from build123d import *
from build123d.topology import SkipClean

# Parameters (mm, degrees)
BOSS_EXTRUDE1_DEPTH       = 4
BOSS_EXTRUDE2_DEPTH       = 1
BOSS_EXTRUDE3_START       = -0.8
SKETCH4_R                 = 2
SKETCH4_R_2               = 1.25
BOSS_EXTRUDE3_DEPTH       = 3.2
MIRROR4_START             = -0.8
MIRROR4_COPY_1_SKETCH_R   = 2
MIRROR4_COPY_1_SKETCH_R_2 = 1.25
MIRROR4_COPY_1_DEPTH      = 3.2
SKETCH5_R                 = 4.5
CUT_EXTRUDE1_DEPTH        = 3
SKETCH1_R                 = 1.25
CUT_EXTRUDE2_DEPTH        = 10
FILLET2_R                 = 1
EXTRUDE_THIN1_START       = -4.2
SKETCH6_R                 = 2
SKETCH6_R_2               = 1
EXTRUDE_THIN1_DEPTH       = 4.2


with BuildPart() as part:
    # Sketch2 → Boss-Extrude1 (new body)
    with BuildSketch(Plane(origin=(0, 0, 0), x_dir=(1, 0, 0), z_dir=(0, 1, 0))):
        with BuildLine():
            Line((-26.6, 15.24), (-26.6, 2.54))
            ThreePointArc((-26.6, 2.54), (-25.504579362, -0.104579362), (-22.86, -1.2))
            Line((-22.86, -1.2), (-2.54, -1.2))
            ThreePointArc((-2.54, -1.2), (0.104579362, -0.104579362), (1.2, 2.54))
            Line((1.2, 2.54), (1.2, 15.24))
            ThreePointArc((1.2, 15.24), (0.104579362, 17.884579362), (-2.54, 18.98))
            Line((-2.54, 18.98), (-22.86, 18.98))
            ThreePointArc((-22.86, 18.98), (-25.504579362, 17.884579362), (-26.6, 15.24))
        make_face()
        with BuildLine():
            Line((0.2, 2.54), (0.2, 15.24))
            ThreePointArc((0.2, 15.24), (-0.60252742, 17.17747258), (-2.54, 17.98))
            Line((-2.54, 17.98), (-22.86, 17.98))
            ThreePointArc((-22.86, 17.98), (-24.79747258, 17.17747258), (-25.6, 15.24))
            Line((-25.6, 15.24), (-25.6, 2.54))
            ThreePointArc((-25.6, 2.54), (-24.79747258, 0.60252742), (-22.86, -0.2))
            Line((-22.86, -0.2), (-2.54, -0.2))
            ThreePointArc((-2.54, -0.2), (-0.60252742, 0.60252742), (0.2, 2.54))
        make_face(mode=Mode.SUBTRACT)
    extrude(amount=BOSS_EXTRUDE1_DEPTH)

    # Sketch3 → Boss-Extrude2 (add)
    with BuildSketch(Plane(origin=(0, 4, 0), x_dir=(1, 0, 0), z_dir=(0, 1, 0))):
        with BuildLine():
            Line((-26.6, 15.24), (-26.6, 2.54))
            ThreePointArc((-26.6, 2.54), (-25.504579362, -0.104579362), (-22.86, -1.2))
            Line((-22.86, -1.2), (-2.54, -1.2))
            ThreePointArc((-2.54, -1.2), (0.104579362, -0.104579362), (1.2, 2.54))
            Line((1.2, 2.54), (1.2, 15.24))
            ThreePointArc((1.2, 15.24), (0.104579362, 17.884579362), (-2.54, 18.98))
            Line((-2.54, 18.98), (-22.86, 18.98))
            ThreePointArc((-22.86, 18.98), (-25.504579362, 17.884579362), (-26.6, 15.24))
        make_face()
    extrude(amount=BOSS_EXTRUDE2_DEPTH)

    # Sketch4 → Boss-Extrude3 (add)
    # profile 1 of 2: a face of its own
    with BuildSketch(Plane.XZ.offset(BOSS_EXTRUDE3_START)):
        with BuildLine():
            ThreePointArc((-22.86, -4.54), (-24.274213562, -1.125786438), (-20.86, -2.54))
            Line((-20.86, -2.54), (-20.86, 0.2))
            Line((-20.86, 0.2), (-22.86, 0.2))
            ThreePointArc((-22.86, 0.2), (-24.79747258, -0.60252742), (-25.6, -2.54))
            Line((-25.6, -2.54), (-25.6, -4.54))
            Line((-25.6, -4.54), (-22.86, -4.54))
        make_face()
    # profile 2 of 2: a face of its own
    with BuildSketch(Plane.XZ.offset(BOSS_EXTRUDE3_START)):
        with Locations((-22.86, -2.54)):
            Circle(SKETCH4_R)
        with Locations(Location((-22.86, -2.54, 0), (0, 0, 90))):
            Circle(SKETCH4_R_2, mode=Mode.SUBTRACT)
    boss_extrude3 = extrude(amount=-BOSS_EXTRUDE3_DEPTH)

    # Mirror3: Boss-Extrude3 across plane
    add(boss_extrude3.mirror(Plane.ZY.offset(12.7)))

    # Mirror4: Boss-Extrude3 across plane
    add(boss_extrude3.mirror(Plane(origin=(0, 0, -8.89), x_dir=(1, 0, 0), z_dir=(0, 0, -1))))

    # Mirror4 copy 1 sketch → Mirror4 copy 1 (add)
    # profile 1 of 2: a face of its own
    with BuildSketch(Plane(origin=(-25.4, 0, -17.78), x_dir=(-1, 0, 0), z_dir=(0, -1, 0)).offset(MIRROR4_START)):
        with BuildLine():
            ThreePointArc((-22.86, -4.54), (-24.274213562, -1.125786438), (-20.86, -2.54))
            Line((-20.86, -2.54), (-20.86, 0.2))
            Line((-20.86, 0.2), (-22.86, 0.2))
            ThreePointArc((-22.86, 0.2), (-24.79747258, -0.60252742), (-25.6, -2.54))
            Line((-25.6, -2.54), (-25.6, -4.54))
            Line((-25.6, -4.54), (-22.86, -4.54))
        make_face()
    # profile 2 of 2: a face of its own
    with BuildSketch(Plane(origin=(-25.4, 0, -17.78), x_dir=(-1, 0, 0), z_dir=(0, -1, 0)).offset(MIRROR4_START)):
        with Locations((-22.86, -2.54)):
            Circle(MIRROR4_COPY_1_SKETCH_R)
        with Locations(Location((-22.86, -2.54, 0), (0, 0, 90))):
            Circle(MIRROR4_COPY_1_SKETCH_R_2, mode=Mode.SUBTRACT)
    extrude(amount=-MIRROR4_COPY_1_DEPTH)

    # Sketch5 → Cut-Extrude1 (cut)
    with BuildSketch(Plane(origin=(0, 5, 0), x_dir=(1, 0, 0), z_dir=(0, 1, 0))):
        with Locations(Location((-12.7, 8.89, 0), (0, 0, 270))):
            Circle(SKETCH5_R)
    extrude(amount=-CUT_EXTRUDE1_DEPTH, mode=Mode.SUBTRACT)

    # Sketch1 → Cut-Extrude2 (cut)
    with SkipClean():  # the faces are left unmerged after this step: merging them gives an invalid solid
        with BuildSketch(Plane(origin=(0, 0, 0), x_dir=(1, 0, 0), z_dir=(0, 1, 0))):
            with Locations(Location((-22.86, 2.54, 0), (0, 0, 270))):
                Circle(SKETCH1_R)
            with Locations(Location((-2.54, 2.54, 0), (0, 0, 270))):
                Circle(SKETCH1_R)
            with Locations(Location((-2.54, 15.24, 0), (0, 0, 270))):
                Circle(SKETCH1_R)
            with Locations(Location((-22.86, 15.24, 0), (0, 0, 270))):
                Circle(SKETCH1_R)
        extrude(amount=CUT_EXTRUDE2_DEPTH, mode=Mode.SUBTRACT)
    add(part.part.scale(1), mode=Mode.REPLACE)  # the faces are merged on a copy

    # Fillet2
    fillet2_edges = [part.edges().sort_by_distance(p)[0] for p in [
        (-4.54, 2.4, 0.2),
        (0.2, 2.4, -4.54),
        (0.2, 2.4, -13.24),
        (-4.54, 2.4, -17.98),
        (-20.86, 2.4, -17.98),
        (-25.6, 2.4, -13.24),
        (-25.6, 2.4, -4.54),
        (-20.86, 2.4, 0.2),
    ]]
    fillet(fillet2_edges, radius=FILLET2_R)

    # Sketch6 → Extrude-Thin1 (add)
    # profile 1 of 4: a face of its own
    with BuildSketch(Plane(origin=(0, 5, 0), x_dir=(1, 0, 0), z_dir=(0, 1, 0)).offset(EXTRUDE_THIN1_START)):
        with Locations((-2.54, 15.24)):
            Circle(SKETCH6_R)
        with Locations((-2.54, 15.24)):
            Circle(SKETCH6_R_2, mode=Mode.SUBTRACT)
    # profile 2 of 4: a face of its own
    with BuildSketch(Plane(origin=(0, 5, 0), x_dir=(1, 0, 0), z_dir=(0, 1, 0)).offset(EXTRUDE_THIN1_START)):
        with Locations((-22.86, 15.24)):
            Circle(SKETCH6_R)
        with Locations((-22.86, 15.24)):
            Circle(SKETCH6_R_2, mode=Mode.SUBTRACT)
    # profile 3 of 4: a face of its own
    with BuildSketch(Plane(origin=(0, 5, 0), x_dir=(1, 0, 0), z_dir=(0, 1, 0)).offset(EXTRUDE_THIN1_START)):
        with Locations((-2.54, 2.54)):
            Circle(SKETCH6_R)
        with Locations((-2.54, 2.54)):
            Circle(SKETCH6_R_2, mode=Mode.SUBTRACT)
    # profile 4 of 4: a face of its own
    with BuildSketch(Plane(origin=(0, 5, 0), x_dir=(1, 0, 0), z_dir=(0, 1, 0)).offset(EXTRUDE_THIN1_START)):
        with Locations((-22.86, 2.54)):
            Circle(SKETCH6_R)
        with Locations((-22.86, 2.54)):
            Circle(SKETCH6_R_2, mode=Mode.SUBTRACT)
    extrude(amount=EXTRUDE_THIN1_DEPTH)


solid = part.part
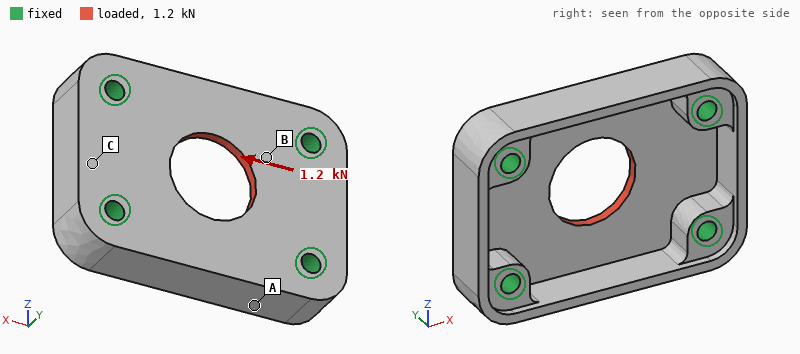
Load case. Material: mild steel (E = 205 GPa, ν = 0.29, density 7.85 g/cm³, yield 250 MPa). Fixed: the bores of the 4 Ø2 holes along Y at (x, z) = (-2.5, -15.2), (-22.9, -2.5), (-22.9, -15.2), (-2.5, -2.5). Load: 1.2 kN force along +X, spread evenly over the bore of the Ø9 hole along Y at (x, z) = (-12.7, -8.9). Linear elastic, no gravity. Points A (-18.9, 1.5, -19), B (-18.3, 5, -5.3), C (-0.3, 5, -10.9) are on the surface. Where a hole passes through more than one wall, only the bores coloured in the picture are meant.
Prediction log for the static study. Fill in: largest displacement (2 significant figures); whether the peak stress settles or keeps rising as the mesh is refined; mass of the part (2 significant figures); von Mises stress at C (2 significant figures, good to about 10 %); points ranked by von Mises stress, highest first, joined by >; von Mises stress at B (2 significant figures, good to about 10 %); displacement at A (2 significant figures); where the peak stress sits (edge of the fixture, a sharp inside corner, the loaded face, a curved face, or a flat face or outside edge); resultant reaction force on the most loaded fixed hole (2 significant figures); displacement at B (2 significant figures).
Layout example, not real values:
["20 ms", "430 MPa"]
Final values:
["1.8 µm", "keeps rising", "8.2 g", "17 MPa", "B > C > A", "42 MPa", "0.32 µm", "edge of the fixture", "310 N", "1.2 µm"]
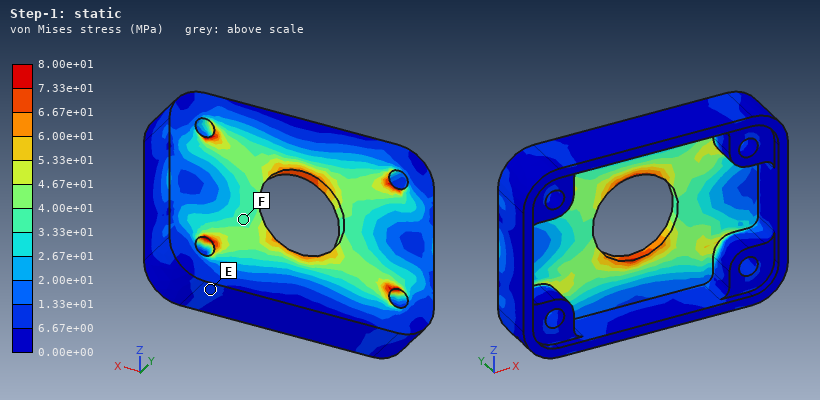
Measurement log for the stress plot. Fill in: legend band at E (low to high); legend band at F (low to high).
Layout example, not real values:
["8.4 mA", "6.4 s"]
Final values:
["6.67e+00 to 1.33e+01 MPa", "3.33e+01 to 4.00e+01 MPa"]
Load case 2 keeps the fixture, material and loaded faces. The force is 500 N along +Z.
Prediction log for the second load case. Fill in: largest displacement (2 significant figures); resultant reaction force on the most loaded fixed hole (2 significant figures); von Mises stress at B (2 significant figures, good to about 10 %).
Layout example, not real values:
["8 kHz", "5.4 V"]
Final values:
["1.8 µm", "140 N", "21 MPa"]
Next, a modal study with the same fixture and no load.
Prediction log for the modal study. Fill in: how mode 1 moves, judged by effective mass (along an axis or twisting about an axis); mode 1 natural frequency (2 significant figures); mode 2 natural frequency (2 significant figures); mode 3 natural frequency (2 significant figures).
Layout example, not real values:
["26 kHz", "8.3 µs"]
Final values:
["along Y", "23 kHz", "30 kHz", "35 kHz"]
